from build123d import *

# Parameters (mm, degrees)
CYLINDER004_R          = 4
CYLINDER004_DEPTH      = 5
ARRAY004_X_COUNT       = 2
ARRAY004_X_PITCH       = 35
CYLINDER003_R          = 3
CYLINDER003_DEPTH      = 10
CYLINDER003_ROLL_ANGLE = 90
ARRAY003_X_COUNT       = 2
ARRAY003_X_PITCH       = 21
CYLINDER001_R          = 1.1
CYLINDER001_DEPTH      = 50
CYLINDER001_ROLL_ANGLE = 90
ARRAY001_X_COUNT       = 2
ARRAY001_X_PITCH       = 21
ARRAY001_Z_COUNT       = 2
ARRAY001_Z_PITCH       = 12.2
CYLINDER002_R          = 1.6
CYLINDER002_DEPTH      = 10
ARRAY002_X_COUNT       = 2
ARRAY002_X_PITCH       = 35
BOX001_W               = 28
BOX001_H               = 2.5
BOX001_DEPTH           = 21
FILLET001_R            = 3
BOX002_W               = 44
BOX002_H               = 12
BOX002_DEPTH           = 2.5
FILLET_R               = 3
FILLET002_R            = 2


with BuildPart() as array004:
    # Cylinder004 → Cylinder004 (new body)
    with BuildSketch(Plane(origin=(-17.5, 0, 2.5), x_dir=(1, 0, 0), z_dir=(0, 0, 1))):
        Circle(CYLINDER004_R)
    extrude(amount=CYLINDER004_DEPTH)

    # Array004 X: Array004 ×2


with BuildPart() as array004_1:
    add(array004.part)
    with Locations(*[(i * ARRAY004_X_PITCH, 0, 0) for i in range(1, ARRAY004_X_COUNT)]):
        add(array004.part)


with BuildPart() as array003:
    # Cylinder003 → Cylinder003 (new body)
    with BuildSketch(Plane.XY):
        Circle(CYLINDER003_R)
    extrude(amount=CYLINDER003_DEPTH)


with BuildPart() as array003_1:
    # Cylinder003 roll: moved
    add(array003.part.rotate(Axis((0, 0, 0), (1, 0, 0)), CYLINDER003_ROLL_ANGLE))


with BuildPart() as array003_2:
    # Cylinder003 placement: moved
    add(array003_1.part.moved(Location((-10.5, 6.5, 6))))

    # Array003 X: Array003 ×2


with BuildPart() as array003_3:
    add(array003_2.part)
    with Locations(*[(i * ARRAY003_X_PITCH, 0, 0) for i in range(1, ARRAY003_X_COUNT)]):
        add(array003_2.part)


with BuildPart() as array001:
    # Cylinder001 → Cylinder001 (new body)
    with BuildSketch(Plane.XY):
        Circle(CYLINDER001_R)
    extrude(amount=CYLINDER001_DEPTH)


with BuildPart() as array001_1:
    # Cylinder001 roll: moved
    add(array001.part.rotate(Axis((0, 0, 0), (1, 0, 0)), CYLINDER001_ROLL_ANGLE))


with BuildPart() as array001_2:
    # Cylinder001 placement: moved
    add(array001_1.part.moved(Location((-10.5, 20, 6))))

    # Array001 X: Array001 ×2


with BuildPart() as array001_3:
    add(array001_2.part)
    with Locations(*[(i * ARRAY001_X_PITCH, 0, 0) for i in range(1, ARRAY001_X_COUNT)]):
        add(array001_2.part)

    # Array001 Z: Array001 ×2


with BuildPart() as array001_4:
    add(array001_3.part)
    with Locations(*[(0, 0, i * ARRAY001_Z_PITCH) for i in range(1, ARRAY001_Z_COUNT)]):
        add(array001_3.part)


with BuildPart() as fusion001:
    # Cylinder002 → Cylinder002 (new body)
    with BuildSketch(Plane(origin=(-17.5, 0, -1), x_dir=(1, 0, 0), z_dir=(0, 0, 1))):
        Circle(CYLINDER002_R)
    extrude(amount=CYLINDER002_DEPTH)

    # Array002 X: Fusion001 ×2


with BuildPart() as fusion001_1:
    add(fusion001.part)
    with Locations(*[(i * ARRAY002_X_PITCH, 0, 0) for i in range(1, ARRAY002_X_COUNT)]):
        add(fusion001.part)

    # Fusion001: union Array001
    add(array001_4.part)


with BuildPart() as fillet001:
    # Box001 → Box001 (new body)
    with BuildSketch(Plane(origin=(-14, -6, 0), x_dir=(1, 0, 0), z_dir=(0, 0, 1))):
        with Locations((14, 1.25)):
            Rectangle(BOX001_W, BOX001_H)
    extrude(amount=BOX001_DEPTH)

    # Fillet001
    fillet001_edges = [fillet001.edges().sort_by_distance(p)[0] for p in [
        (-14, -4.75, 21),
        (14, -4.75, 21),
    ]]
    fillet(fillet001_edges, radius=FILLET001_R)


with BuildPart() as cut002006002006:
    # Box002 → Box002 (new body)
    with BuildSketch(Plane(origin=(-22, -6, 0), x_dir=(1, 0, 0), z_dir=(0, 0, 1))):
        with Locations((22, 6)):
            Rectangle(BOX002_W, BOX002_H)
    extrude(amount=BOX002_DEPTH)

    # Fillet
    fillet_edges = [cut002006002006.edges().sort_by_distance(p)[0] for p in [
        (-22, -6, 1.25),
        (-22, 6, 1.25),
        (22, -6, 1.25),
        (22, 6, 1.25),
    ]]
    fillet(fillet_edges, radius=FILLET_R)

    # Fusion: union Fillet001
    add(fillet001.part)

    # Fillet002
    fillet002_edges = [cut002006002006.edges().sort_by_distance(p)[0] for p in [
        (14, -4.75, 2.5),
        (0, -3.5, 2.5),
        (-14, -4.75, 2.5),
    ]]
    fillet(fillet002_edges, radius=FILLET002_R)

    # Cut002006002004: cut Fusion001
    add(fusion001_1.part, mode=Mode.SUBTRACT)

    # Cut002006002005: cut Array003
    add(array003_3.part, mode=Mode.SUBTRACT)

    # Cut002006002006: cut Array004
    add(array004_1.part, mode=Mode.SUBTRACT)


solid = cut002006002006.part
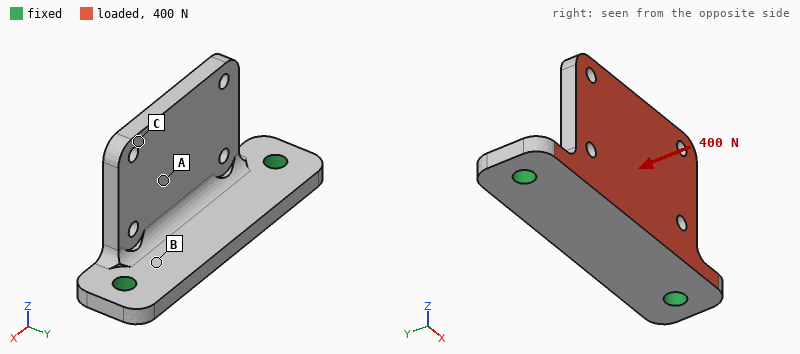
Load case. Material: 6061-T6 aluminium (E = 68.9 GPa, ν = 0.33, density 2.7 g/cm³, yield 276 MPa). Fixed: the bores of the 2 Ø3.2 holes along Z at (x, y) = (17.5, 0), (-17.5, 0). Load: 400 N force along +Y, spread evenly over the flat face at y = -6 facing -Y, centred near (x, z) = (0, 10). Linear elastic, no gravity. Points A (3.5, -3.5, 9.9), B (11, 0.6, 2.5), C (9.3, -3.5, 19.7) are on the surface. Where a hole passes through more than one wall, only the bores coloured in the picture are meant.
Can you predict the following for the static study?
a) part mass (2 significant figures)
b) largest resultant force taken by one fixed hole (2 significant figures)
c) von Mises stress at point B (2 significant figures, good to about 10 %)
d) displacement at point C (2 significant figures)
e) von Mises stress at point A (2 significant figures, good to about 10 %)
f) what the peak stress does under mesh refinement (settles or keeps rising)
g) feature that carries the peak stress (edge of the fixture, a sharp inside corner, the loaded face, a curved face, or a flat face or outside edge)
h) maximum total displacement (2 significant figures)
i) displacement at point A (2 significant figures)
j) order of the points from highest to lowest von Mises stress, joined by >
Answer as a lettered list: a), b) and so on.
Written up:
a) 6.8 g
b) 200 N
c) 74 MPa
d) 0.25 mm
e) 40 MPa
f) keeps rising
g) edge of the fixture
h) 0.27 mm
i) 0.10 mm
j) B > A > C
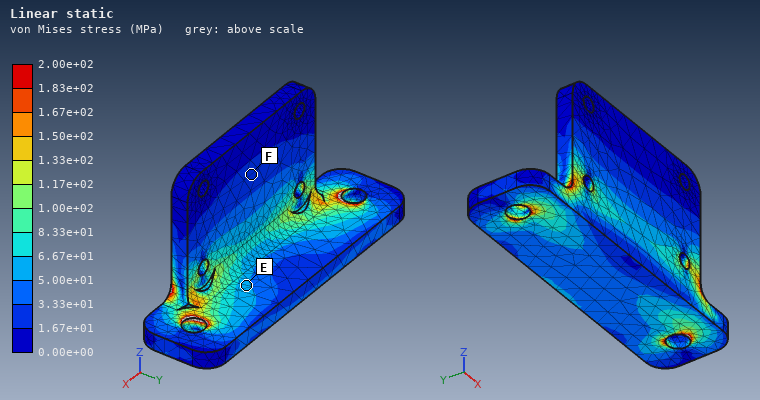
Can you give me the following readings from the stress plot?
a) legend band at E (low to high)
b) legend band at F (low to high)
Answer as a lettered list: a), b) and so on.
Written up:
a) 5.00e+01 to 6.67e+01 MPa
b) 1.67e+01 to 3.33e+01 MPa
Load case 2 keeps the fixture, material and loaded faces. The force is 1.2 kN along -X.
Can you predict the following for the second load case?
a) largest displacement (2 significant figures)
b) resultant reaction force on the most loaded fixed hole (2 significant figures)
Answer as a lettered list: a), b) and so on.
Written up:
a) 34 µm
b) 720 N
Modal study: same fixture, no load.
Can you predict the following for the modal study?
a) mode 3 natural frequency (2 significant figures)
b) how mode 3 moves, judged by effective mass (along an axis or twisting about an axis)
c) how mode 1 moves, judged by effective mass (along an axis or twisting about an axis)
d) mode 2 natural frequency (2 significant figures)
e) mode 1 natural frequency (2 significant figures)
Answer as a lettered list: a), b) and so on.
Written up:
a) 13 kHz
b) along Z
c) along Y
d) 9400 Hz
e) 3700 Hz
